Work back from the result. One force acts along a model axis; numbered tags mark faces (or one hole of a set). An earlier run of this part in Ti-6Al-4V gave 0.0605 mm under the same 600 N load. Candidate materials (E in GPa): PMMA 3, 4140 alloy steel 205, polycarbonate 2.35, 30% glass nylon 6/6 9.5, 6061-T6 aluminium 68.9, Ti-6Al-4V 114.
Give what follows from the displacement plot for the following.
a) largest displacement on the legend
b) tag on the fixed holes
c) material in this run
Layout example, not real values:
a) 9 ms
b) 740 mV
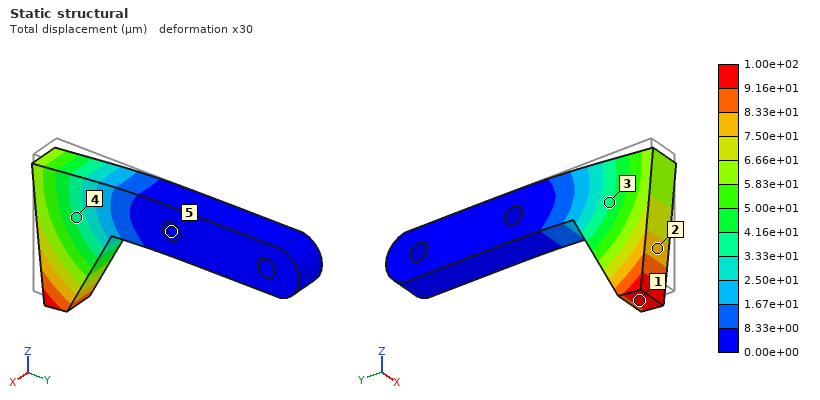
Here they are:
a) 1.00e+02 µm
b) 5
c) 6061-T6 aluminium
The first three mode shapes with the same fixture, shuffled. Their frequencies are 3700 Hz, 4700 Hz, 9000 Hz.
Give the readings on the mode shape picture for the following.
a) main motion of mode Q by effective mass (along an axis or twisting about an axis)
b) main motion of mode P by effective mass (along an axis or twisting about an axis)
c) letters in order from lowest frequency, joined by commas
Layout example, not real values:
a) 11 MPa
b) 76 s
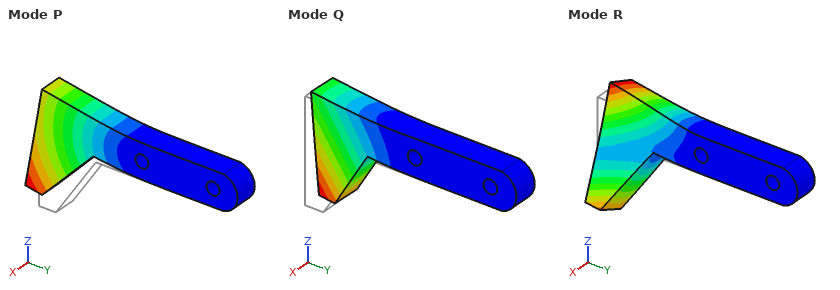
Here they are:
a) along X
b) along Z
c) Q, P, R
